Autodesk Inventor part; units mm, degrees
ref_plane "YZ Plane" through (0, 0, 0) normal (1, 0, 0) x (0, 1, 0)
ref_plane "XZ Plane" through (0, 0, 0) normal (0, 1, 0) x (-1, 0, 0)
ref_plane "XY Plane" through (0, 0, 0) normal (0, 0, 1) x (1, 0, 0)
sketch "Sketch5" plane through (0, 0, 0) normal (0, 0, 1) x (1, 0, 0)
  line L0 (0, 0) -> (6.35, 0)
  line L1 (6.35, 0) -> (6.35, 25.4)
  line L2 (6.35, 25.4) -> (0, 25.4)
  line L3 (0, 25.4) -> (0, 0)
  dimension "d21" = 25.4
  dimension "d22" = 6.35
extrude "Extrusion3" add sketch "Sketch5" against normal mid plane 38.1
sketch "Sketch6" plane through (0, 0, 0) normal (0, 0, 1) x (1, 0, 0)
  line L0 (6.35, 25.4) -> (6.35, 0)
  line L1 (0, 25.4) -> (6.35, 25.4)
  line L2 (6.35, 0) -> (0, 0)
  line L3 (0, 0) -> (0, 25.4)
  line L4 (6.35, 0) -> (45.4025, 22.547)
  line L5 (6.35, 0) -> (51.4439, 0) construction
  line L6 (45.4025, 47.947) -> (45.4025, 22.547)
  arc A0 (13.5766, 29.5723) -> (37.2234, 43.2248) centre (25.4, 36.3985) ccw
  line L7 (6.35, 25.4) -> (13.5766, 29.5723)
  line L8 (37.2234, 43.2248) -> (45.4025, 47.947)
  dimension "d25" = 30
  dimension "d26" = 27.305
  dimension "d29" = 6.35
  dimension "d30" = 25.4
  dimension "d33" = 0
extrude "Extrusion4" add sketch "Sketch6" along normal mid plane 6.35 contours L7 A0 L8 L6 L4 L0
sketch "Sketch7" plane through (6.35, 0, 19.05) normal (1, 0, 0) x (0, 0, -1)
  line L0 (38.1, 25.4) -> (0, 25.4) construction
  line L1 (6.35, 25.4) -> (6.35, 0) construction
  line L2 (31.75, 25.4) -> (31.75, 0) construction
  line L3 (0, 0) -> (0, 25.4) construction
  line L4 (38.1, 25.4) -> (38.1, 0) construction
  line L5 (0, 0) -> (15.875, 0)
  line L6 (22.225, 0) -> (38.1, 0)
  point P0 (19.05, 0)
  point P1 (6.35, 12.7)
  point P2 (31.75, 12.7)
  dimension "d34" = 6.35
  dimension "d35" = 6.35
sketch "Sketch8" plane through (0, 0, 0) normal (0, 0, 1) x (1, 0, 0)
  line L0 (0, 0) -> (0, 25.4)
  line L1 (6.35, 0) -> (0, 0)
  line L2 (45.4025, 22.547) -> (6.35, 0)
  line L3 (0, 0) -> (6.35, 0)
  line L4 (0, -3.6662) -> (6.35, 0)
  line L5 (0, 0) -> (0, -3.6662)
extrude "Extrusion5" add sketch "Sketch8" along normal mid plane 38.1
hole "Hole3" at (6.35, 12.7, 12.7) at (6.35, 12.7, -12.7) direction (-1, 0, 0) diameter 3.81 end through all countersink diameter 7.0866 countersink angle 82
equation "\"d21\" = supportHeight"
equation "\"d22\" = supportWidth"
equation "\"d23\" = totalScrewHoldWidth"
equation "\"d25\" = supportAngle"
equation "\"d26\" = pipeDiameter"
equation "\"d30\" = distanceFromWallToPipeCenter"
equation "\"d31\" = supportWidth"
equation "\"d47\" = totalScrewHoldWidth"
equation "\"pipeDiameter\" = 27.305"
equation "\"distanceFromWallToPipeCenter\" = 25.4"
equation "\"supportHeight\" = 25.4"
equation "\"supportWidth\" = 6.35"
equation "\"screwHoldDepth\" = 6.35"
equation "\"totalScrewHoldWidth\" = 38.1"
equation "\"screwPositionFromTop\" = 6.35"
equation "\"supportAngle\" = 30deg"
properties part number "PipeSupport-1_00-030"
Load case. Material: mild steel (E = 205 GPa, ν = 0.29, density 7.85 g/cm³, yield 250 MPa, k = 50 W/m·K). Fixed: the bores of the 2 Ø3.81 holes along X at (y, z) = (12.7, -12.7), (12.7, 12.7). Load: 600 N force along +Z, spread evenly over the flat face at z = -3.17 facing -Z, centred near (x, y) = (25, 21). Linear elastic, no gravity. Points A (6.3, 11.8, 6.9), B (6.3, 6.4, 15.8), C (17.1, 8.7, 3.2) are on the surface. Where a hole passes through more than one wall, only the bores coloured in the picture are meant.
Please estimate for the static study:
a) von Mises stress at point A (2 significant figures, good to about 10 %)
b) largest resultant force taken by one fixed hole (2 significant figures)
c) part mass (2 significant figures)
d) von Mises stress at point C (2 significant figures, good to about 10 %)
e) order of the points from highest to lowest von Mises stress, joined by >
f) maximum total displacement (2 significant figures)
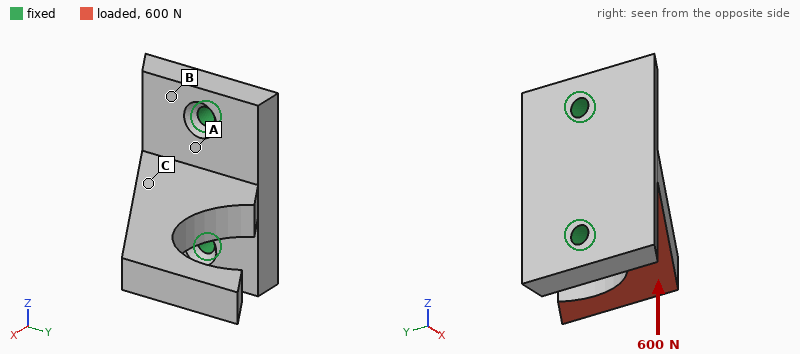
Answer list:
17 MPa
690 N
85 g
53 MPa
C > A > B
0.13 mm
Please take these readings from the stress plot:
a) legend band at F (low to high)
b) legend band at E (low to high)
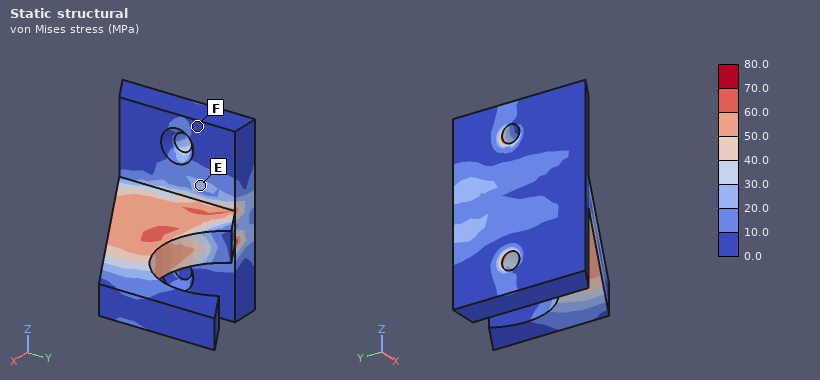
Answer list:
0.0 to 10.0 MPa
20.0 to 30.0 MPa
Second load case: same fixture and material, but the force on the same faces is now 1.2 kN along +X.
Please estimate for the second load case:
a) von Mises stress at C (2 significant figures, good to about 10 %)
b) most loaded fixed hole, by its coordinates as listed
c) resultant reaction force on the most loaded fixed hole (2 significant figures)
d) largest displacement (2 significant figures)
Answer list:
27 MPa
(12.7, -12.7)
820 N
82 µm
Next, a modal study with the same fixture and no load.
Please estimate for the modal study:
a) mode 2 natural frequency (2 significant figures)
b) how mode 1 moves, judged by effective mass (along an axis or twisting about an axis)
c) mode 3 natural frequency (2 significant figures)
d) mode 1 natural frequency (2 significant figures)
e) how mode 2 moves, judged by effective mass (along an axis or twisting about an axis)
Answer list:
3300 Hz
along Z
7300 Hz
2400 Hz
along Y
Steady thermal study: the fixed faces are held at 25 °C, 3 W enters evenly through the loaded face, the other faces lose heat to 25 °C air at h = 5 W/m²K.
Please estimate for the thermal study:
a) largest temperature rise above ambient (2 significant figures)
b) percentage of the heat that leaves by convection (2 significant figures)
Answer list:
18 K
3.4 %
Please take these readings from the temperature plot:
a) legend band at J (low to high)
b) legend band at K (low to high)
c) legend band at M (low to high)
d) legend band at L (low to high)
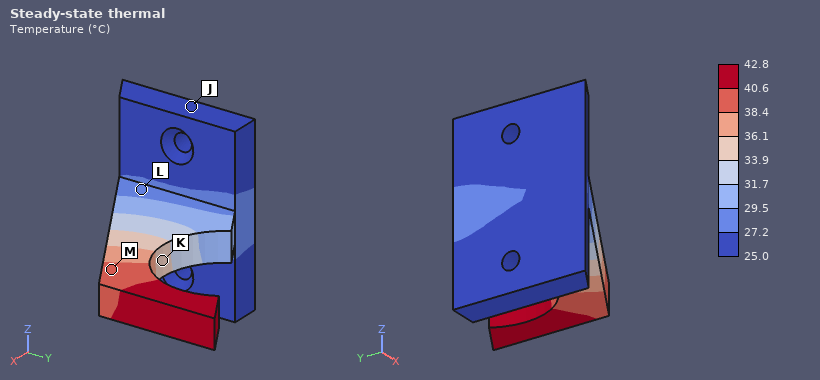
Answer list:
25.0 to 27.2 °C
33.9 to 36.1 °C
38.4 to 40.6 °C
27.2 to 29.5 °C
